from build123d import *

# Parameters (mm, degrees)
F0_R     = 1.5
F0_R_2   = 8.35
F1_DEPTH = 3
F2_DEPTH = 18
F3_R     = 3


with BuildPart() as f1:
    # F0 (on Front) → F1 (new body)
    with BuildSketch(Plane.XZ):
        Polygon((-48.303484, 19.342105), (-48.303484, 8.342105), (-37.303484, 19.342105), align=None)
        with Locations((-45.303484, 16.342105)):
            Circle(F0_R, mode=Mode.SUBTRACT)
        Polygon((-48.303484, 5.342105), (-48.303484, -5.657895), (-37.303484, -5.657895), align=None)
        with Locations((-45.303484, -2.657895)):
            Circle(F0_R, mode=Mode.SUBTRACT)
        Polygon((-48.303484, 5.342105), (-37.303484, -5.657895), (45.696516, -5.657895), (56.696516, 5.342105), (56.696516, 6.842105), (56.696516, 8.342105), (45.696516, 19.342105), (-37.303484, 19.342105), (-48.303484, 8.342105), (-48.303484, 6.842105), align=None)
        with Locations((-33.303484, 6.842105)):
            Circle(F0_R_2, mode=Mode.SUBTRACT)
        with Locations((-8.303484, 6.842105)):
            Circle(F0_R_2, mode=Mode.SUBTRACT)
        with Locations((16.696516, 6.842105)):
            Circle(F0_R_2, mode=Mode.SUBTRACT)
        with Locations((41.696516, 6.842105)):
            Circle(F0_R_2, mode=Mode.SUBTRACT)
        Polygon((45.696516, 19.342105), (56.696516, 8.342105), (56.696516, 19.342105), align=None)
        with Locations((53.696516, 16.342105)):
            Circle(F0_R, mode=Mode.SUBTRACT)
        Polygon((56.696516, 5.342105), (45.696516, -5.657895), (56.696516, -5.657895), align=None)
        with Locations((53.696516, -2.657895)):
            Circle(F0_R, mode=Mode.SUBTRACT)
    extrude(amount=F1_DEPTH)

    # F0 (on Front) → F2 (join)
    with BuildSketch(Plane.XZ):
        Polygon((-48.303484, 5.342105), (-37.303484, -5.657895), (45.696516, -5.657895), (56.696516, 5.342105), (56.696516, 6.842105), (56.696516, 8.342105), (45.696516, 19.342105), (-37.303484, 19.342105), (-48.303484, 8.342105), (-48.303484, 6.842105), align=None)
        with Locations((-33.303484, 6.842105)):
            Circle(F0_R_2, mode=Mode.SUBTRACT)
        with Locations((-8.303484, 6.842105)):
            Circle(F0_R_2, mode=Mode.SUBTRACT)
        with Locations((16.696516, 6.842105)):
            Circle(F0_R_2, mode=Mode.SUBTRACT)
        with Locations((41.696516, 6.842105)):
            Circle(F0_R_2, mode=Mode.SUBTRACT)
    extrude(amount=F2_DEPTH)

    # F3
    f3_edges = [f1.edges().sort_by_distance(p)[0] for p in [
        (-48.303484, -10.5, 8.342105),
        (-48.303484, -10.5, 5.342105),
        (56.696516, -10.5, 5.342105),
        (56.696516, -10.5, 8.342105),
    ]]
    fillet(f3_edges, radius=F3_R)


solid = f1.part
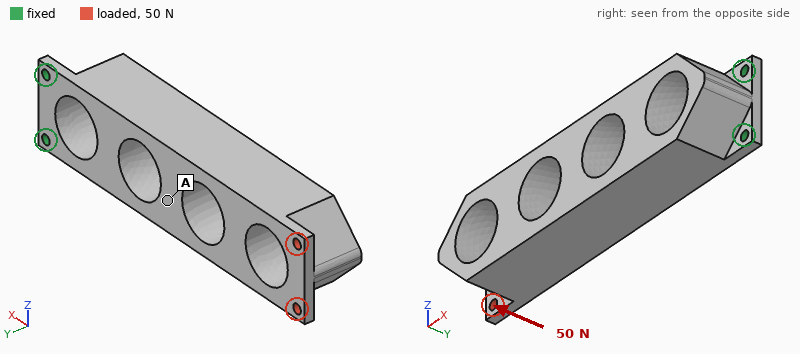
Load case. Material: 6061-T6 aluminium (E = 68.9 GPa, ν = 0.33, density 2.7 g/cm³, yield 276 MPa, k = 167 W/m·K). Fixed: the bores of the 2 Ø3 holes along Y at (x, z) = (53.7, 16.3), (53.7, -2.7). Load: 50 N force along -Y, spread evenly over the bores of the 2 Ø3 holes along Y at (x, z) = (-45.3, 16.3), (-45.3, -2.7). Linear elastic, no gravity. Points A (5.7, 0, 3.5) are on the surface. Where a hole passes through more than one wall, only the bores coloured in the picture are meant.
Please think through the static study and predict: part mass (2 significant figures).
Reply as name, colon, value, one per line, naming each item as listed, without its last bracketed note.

part mass: 75 g
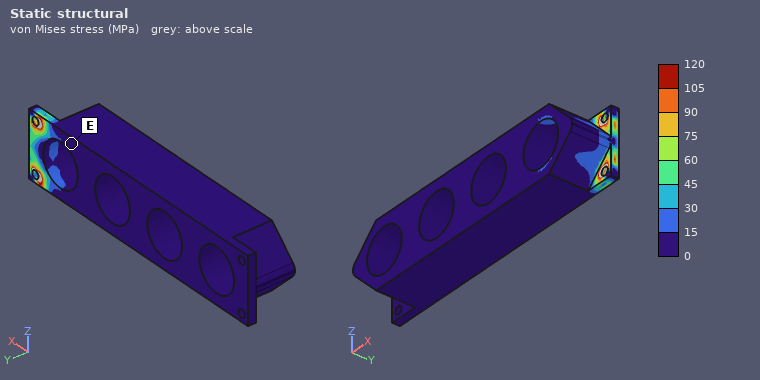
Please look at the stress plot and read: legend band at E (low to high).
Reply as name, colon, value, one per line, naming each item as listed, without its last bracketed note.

legend band at E: 0 to 15 MPa
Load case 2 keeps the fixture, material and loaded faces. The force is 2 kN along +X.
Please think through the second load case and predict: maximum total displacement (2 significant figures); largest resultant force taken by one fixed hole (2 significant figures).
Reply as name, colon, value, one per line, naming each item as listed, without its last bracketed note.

maximum total displacement: 0.25 mm
largest resultant force taken by one fixed hole: 1.0 kN
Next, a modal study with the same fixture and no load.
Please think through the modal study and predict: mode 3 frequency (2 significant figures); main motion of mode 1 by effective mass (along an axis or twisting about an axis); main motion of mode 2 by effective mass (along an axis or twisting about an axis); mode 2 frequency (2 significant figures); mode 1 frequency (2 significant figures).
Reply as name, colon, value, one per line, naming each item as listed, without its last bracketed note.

mode 3 frequency: 3600 Hz
main motion of mode 1 by effective mass: along Y
main motion of mode 2 by effective mass: along Z
mode 2 frequency: 1200 Hz
mode 1 frequency: 320 Hz
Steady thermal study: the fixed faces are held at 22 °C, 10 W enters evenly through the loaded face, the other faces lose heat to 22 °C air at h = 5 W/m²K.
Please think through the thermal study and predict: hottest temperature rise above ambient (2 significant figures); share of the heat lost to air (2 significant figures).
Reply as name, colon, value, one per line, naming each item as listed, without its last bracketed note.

hottest temperature rise above ambient: 39 K
share of the heat lost to air: 10 %
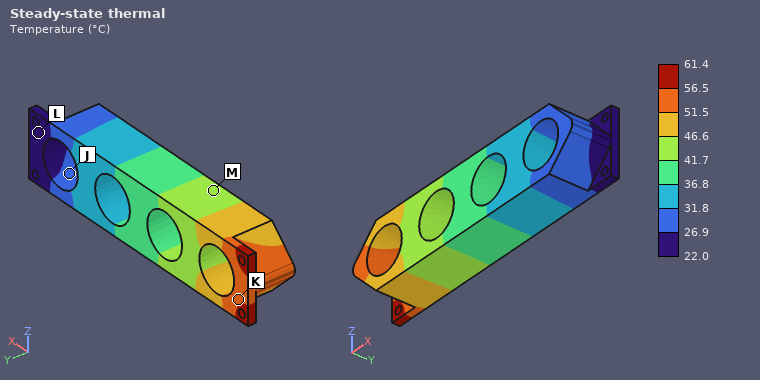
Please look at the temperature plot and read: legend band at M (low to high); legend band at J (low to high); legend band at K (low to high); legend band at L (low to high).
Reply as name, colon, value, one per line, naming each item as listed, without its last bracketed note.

legend band at M: 41.7 to 46.6 °C
legend band at J: 26.9 to 31.8 °C
legend band at K: 51.5 to 56.5 °C
legend band at L: 22.0 to 26.9 °C
